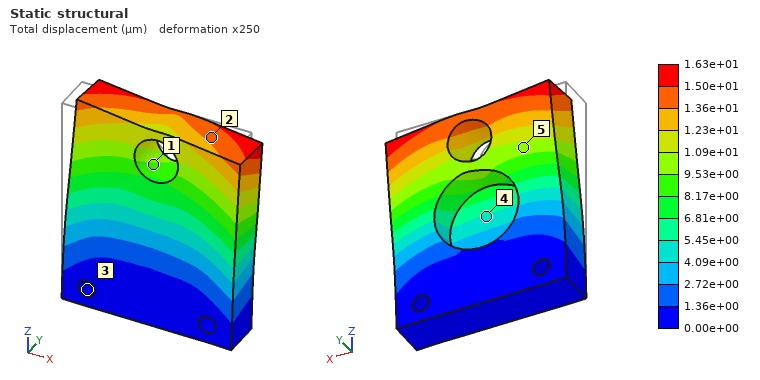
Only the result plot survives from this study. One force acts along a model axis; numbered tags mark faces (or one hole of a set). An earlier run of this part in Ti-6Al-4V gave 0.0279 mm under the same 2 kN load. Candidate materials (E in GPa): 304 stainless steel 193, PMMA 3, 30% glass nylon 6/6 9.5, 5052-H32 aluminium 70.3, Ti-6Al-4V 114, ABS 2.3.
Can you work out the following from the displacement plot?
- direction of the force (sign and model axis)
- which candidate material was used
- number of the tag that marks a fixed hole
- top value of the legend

+X
304 stainless steel
3
1.63e+01 µm
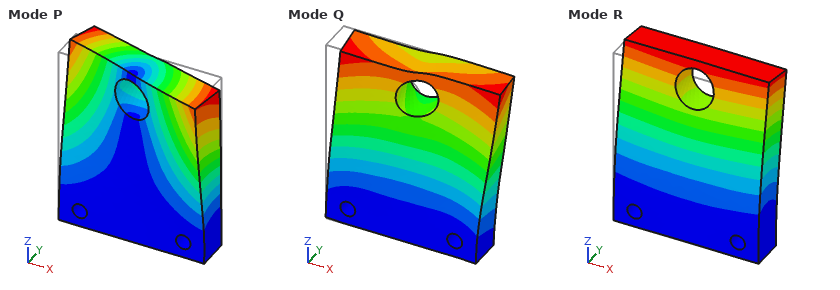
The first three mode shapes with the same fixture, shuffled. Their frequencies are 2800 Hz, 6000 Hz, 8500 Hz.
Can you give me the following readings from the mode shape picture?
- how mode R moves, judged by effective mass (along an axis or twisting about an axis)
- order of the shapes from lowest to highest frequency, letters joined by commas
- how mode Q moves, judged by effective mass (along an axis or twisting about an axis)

along Y
R, P, Q
along X
